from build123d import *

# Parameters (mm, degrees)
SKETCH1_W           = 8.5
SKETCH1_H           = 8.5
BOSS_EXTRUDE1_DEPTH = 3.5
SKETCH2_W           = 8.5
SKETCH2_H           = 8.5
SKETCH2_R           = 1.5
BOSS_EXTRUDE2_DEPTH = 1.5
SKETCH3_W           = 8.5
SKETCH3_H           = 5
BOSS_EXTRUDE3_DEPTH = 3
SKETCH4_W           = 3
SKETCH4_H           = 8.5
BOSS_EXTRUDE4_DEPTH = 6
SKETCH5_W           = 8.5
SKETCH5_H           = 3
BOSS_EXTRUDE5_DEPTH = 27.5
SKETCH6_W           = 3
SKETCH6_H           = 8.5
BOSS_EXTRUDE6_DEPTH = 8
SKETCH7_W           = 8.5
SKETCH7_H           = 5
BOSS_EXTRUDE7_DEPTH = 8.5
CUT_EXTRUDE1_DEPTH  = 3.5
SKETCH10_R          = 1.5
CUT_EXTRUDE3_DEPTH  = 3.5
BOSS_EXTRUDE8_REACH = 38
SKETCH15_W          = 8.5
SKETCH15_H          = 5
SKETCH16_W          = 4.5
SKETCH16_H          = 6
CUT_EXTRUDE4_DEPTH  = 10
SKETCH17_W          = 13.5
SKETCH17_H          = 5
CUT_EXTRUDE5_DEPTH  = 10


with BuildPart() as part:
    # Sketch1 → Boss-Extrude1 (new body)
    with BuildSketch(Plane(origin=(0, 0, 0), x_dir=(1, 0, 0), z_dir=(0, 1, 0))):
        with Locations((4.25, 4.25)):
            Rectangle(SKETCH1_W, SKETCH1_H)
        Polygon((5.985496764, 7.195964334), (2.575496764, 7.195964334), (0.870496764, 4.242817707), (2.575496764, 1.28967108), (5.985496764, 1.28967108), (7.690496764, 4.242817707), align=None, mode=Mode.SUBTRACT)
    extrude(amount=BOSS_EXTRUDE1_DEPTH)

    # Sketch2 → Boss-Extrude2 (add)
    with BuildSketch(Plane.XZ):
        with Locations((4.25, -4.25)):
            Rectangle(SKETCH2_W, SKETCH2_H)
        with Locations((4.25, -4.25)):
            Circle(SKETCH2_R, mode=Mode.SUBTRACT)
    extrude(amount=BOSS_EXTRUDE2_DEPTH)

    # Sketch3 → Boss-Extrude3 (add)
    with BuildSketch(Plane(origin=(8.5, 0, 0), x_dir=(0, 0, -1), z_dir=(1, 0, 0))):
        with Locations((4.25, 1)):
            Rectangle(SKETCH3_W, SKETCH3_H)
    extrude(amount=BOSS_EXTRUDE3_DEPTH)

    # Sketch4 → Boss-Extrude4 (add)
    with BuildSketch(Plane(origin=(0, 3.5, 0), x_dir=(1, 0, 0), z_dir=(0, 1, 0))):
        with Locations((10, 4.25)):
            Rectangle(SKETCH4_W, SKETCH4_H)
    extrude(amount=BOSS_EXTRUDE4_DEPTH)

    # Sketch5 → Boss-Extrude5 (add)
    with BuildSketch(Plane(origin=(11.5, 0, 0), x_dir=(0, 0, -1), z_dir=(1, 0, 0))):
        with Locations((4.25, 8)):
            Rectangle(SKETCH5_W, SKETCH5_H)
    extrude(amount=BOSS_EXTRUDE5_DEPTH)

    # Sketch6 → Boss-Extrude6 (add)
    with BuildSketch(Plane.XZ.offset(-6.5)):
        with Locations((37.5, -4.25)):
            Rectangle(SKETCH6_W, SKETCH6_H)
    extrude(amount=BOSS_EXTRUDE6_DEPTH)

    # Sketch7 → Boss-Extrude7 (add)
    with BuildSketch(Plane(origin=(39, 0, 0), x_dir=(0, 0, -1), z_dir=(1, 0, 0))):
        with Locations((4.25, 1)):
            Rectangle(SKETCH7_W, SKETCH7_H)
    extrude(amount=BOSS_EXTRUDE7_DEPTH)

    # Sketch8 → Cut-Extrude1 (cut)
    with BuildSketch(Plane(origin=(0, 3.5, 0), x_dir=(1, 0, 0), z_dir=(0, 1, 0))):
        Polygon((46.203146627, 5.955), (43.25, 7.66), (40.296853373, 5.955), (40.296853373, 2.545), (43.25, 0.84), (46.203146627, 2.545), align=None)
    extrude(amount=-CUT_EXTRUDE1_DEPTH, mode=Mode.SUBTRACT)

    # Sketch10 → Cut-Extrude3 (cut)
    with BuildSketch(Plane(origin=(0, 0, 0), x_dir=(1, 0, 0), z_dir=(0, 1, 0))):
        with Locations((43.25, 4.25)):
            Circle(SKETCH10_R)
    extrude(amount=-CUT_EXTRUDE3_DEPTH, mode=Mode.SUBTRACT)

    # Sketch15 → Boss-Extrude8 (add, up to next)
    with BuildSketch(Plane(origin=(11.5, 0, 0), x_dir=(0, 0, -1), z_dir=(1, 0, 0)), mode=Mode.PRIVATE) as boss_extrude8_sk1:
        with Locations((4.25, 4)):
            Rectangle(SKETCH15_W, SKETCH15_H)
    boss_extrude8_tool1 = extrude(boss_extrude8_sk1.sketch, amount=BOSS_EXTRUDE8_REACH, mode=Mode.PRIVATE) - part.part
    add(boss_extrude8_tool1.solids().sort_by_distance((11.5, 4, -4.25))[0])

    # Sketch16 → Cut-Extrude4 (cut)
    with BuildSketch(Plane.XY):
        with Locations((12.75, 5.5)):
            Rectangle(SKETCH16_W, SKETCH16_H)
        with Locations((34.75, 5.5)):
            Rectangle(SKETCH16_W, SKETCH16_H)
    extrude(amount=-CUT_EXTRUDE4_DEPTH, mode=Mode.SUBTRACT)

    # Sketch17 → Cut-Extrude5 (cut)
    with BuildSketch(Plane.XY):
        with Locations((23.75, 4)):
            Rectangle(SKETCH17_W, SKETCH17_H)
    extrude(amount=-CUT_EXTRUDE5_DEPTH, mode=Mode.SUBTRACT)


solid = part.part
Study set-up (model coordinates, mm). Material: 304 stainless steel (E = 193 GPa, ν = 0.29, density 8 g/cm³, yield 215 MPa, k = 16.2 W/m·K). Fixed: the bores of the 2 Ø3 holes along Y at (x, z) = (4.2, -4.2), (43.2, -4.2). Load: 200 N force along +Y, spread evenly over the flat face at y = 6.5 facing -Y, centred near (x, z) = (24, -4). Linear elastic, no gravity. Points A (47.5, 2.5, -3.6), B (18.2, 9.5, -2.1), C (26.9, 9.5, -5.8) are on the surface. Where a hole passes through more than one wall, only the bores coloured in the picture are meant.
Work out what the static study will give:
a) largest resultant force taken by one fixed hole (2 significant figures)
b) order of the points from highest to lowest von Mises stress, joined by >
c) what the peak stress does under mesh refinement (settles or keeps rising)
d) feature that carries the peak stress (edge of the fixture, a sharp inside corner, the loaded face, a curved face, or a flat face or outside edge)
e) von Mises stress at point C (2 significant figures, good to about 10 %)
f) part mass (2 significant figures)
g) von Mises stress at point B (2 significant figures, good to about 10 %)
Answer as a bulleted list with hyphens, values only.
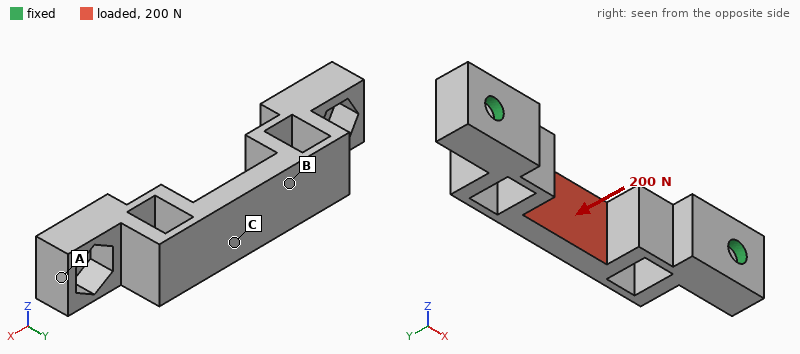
- 160 N
- C > B > A
- keeps rising
- edge of the fixture
- 19 MPa
- 13 g
- 9.3 MPa
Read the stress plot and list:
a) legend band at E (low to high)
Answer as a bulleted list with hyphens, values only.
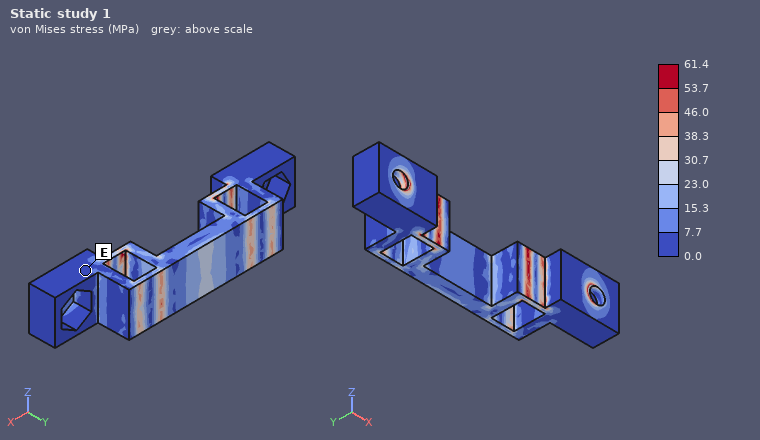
- 0.0 to 7.7 MPa
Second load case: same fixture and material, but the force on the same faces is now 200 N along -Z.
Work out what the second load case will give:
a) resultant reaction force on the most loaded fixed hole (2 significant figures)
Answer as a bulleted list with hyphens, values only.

- 100 N
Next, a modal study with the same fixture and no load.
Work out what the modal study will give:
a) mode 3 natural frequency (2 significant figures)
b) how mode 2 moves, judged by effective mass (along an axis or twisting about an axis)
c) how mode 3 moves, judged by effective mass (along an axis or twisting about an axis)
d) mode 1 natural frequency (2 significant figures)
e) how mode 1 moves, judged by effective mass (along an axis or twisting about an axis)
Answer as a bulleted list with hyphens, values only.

- 14 kHz
- along Y
- along X
- 8000 Hz
- along Z
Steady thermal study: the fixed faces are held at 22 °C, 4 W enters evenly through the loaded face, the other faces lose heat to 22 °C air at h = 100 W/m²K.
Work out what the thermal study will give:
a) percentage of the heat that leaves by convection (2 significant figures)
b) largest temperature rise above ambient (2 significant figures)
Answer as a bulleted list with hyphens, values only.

- 76 %
- 52 K
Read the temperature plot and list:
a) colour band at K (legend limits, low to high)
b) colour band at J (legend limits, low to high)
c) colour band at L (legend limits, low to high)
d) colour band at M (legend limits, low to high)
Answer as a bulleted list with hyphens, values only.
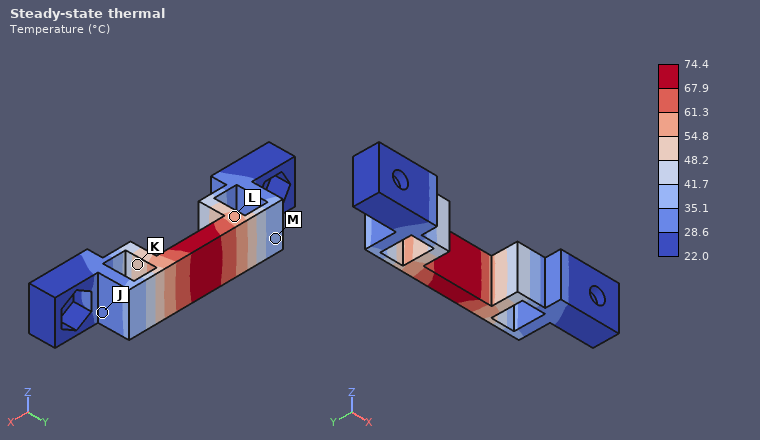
- 48.2 to 54.8 °C
- 28.6 to 35.1 °C
- 54.8 to 61.3 °C
- 35.1 to 41.7 °C
